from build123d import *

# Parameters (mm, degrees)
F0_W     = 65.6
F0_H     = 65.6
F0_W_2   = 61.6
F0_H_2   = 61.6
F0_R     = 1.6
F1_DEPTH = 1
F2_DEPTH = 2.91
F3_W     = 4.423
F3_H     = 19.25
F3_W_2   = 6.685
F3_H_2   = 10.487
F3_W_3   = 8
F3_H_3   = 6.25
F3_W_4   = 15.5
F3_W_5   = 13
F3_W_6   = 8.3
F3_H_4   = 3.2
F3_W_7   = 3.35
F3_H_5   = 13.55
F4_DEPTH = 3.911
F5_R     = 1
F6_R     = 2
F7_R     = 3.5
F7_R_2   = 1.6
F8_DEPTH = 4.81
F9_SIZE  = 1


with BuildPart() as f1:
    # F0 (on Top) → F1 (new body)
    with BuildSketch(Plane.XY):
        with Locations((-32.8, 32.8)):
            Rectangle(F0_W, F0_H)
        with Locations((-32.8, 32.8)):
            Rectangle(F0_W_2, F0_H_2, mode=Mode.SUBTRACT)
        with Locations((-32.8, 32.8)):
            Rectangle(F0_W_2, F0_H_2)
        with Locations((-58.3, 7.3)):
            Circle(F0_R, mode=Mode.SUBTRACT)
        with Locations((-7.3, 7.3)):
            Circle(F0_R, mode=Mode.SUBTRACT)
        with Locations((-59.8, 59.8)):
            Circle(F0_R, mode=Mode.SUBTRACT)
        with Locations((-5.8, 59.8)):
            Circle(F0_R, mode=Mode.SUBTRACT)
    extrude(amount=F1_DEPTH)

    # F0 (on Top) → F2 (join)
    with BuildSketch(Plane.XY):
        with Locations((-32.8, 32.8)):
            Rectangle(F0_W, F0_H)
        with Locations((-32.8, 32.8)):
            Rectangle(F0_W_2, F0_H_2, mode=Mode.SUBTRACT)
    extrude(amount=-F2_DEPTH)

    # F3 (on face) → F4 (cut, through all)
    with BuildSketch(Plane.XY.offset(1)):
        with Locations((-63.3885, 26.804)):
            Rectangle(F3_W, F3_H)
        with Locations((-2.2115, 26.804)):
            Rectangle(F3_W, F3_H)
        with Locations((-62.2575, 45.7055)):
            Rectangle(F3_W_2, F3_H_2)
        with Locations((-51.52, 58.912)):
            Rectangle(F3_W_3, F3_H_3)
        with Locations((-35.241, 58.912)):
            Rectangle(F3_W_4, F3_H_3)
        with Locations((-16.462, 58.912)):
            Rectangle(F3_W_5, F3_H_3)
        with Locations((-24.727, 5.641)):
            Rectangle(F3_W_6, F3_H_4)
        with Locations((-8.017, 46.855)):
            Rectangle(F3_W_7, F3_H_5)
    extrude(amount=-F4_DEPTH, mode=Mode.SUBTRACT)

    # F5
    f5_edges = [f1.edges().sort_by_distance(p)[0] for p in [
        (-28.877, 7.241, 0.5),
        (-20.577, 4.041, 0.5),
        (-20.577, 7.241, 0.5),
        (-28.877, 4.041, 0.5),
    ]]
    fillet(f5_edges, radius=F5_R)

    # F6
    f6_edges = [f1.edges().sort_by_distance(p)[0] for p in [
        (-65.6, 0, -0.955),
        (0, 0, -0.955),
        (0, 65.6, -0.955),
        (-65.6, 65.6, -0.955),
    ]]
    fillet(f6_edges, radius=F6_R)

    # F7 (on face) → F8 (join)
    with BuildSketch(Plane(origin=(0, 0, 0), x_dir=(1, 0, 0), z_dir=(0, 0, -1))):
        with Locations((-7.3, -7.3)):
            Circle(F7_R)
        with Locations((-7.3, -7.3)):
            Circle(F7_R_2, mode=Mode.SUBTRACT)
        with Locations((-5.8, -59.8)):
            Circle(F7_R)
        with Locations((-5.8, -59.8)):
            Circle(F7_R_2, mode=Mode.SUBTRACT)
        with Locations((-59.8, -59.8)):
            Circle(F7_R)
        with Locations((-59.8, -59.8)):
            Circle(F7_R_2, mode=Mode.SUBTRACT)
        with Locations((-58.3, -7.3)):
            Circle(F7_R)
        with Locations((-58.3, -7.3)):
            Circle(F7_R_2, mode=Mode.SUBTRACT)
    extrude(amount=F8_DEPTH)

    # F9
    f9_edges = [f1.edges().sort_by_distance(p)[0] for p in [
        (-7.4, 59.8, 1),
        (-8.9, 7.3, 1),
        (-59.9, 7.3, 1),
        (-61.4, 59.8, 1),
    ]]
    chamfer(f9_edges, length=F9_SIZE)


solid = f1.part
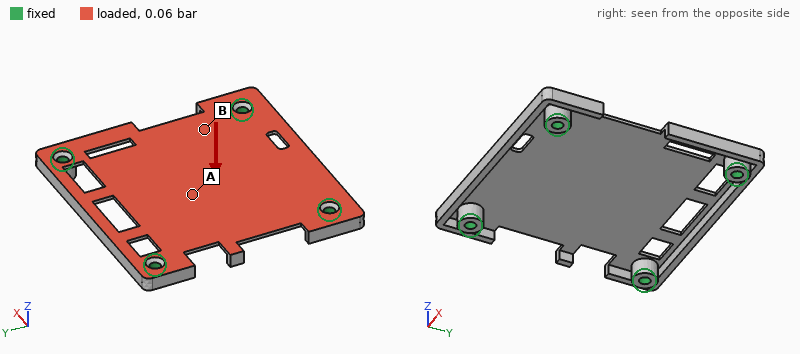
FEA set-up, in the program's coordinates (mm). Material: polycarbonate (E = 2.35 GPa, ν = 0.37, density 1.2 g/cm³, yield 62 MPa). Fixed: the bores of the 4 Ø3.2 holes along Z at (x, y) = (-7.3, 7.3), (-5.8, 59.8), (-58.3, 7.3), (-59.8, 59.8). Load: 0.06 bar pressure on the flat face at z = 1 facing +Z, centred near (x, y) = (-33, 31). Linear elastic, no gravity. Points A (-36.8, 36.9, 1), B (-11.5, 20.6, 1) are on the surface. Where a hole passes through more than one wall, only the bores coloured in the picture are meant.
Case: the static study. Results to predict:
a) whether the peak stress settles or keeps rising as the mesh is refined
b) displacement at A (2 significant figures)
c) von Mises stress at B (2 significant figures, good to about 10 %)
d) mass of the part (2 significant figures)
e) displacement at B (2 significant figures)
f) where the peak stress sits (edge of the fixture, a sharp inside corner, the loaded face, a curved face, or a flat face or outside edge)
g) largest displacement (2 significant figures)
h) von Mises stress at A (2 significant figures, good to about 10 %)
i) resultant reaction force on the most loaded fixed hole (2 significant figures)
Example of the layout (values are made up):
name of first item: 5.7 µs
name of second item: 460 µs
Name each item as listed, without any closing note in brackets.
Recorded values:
whether the peak stress settles or keeps rising as the mesh is refined: keeps rising
displacement at A: 0.98 mm
von Mises stress at B: 1.5 MPa
mass of the part: 6.6 g
displacement at B: 0.31 mm
where the peak stress sits: a sharp inside corner
largest displacement: 0.99 mm
von Mises stress at A: 4.8 MPa
resultant reaction force on the most loaded fixed hole: 7.0 N
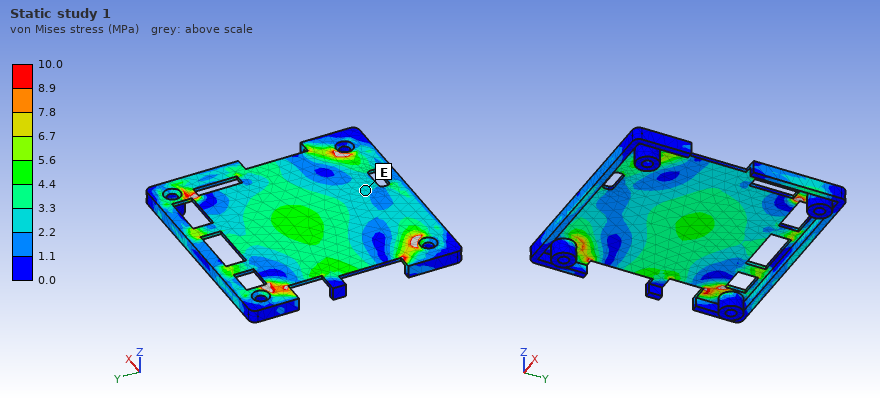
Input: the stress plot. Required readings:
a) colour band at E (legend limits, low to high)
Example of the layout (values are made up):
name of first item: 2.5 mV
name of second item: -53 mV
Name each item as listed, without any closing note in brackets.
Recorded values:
colour band at E: 2.2 to 3.3 MPa
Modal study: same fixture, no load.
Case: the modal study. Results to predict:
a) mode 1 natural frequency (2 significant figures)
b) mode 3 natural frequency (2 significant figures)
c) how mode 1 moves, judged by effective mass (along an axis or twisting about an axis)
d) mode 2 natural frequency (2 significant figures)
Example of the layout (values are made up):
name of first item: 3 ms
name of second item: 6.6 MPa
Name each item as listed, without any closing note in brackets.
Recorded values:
mode 1 natural frequency: 440 Hz
mode 3 natural frequency: 970 Hz
how mode 1 moves, judged by effective mass: along Z
mode 2 natural frequency: 700 Hz
